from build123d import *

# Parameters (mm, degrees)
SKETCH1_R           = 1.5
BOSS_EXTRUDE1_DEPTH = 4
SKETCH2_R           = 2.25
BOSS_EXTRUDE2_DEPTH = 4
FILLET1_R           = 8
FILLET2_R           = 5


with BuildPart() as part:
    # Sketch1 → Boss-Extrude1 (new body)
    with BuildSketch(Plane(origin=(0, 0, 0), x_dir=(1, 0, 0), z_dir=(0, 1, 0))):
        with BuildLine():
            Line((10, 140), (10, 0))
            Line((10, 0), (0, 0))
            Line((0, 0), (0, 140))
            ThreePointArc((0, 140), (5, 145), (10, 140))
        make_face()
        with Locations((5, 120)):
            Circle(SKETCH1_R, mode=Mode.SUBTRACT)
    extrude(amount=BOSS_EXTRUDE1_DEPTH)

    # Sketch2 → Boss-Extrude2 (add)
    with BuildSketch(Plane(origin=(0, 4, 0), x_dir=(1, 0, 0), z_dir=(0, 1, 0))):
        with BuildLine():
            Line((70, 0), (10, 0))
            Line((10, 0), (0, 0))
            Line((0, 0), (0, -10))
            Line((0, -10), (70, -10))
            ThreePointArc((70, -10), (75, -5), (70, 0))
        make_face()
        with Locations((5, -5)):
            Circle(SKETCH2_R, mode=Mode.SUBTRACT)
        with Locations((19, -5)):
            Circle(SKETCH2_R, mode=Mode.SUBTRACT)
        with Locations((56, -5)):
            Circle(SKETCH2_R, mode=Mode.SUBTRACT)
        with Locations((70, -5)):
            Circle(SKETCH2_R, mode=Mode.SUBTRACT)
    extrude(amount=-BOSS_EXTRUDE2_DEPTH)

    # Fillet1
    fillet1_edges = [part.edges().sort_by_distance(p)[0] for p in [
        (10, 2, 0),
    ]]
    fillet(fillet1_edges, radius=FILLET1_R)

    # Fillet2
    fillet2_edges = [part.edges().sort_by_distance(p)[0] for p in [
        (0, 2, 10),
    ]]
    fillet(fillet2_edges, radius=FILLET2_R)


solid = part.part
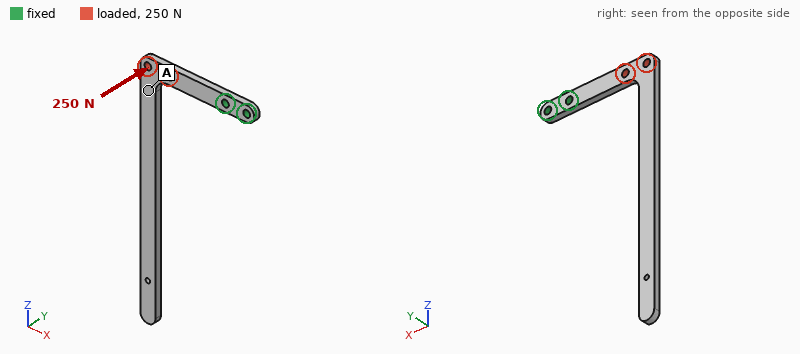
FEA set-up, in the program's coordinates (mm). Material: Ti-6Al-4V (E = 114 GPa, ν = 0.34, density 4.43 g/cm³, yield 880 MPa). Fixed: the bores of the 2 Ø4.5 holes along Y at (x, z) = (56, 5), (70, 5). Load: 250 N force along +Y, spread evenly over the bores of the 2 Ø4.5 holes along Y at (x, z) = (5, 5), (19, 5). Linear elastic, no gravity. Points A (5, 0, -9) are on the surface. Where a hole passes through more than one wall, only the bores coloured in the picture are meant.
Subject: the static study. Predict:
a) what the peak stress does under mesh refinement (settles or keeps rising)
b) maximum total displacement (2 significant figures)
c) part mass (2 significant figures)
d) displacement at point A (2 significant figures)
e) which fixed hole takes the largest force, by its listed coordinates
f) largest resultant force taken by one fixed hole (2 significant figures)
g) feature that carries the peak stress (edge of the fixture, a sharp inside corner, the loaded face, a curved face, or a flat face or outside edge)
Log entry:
keeps rising
1.5 mm
37 g
1.3 mm
(56, 5)
280 N
edge of the fixture
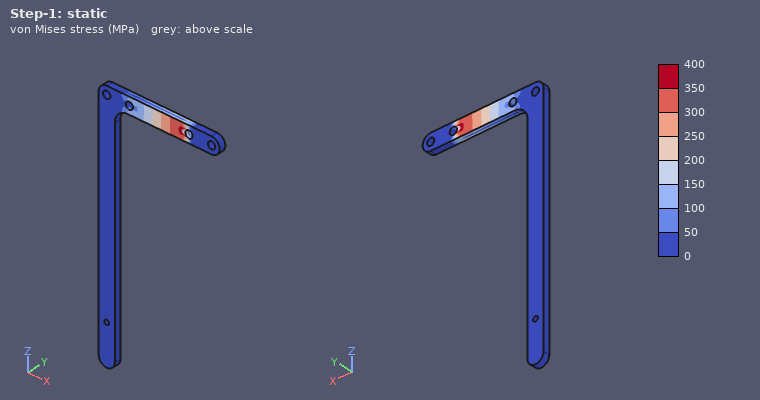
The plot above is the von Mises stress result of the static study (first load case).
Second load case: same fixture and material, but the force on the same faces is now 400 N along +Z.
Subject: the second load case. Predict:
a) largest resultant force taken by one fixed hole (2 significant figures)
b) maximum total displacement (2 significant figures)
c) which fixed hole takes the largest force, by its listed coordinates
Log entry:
720 N
1.7 mm
(56, 5)
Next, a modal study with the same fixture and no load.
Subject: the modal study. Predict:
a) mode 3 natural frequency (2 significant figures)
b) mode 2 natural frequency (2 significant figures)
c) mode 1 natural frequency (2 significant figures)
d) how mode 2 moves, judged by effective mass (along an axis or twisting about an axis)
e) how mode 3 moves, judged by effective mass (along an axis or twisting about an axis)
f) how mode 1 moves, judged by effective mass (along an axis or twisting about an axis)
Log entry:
520 Hz
240 Hz
100 Hz
along X
along Y
along Y
